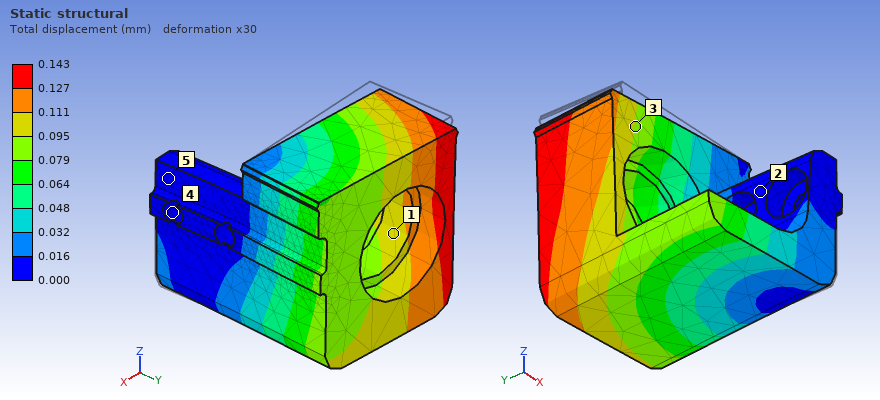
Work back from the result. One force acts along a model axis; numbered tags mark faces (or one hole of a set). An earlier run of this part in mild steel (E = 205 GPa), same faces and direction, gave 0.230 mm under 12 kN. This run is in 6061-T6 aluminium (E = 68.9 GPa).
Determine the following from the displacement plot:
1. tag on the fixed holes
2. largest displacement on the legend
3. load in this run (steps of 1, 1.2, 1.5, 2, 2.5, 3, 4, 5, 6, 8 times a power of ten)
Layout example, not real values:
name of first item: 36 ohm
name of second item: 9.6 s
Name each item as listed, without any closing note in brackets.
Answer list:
tag on the fixed holes: 4
largest displacement on the legend: 0.143 mm
load in this run: 2.5 kN
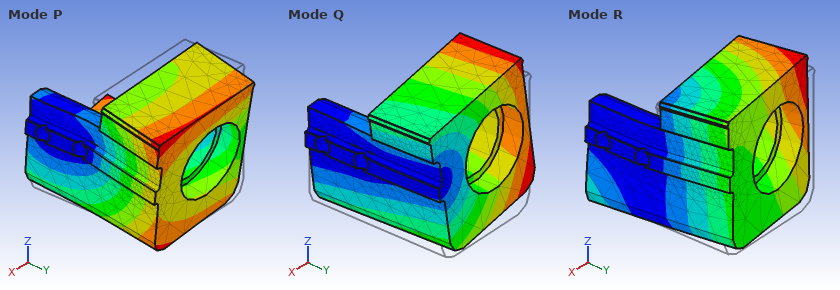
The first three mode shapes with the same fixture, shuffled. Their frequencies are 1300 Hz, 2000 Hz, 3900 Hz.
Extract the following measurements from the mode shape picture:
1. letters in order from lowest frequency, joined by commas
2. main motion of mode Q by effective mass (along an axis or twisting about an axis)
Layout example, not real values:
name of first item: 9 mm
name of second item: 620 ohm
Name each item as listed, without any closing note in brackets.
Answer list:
letters in order from lowest frequency, joined by commas: Q, R, P
main motion of mode Q by effective mass: along Z
